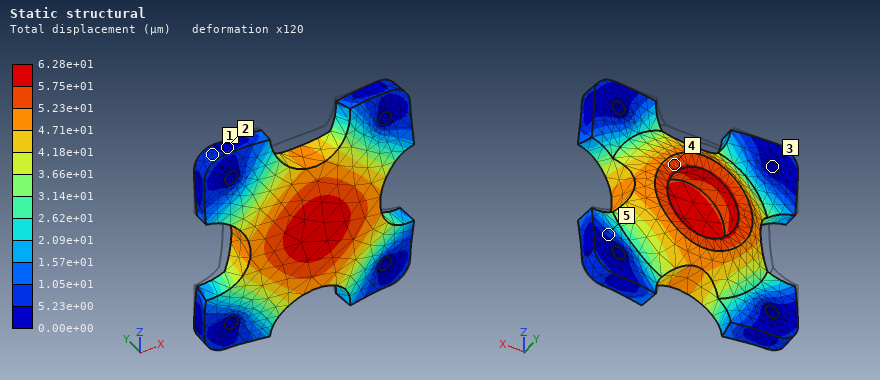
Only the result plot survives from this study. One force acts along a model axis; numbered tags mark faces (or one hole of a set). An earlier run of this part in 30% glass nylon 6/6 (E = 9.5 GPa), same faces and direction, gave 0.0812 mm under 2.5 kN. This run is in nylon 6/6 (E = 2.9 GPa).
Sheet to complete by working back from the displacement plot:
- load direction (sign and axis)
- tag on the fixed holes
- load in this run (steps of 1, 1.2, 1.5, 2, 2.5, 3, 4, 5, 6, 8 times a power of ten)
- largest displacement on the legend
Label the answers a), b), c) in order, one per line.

a) -Y
b) 3
c) 600 N
d) 6.28e+01 µm
